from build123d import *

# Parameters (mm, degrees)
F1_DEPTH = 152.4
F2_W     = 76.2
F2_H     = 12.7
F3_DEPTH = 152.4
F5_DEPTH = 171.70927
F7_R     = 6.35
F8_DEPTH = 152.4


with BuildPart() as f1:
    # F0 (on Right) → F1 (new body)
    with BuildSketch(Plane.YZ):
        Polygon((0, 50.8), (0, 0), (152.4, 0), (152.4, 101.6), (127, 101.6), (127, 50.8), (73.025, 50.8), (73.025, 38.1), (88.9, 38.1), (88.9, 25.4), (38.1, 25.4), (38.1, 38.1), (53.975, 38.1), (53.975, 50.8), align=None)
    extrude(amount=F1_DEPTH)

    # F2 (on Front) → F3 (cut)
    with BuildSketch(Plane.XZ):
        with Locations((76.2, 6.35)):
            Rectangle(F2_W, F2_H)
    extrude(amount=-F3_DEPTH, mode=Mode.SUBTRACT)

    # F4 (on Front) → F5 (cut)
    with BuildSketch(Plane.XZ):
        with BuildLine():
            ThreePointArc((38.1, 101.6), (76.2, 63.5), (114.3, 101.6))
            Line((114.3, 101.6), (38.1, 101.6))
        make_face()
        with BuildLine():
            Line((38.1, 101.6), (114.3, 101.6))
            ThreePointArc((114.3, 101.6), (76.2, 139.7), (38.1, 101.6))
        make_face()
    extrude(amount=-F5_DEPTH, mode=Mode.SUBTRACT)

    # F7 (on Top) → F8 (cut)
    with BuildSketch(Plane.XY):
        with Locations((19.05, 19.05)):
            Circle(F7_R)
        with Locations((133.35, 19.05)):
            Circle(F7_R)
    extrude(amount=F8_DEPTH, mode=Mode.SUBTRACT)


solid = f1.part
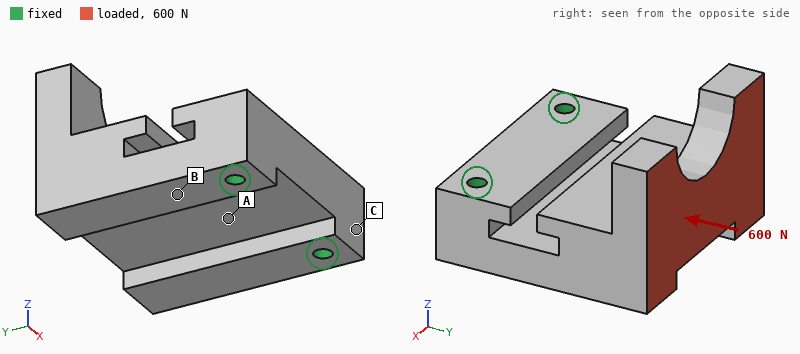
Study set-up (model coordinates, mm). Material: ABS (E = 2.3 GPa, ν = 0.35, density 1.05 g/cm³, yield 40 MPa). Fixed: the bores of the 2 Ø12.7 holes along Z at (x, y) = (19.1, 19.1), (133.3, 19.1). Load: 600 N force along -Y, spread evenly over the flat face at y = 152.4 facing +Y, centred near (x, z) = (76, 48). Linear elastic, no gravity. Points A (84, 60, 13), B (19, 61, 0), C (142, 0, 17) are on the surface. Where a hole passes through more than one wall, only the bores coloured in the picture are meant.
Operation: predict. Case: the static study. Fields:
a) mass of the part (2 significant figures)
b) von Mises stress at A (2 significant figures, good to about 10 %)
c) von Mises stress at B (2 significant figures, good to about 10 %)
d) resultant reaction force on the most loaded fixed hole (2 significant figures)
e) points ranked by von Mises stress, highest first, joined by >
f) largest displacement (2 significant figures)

1.1 kg
0.72 MPa
1.8 MPa
330 N
B > A > C
0.60 mm
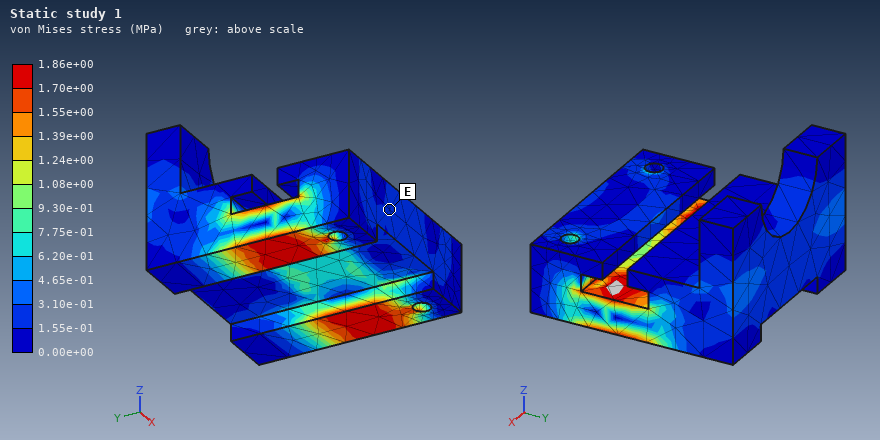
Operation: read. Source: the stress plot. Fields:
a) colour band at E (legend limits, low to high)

1.55e-01 to 3.10e-01 MPa
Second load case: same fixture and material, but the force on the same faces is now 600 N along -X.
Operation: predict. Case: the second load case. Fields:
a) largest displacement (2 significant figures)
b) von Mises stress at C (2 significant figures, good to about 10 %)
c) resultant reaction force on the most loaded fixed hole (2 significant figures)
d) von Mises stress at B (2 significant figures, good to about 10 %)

0.15 mm
0.21 MPa
730 N
0.52 MPa
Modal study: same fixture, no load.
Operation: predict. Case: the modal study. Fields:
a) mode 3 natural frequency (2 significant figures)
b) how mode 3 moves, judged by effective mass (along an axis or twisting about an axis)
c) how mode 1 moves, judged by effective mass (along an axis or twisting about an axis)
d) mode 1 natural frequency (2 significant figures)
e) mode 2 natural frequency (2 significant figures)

710 Hz
along X
along Z
180 Hz
430 Hz
